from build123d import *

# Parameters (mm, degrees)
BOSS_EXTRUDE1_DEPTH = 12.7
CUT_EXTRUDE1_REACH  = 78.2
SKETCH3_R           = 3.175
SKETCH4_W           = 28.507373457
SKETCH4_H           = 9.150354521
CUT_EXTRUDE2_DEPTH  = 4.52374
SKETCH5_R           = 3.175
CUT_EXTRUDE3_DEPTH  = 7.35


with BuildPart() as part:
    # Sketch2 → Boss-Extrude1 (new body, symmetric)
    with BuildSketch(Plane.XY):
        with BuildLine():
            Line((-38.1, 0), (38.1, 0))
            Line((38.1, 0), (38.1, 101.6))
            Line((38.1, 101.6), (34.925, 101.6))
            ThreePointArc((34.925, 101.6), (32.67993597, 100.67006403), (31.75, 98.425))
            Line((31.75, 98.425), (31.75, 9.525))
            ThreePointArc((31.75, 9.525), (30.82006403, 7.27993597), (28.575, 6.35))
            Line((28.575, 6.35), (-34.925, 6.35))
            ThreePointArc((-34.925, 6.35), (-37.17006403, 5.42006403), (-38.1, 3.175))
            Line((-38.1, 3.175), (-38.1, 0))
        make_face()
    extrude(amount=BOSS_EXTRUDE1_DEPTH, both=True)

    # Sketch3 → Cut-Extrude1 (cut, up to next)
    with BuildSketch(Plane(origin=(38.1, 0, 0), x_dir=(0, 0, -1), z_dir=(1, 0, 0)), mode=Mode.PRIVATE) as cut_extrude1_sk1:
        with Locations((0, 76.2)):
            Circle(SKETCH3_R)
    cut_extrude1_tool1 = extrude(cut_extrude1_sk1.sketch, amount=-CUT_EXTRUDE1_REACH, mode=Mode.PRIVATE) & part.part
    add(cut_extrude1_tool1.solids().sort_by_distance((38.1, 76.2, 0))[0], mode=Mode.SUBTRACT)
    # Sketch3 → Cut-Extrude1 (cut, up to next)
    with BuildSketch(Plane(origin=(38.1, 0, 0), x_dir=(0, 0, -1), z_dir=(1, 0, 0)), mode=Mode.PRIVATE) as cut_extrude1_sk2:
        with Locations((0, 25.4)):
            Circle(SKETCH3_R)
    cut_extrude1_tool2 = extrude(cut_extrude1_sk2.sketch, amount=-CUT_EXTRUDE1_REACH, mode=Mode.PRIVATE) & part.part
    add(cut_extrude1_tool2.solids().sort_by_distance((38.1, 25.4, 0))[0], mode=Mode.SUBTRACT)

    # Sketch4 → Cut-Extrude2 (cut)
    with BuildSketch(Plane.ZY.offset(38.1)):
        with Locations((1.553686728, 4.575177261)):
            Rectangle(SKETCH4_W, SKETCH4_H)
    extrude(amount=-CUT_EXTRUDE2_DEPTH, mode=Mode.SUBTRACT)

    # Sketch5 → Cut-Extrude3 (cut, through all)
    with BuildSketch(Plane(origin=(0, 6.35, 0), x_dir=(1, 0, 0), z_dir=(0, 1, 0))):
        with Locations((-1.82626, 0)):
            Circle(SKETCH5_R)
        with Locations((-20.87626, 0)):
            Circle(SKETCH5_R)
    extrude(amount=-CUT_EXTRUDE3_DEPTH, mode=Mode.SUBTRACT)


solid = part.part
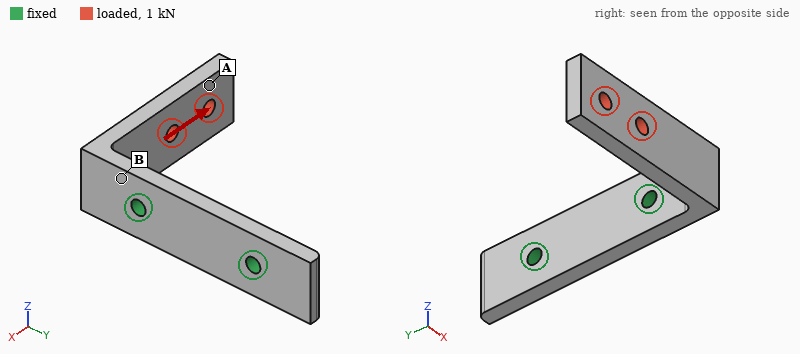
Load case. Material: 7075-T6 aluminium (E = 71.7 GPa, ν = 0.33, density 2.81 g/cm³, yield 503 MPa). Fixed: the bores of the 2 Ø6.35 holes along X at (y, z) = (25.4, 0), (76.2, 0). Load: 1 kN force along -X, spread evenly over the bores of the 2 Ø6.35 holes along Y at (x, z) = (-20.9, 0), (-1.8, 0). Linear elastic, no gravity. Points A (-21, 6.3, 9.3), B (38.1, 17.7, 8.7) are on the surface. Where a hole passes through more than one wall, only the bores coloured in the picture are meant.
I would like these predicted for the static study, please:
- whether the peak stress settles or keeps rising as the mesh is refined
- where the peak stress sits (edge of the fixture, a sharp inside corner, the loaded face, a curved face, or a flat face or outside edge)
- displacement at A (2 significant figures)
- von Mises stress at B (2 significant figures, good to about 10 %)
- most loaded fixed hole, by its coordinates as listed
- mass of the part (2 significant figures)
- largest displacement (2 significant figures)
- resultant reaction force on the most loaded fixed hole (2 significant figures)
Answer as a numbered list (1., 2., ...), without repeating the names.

1. keeps rising
2. edge of the fixture
3. 0.33 mm
4. 71 MPa
5. (25.4, 0)
6. 73 g
7. 0.42 mm
8. 1.0 kN
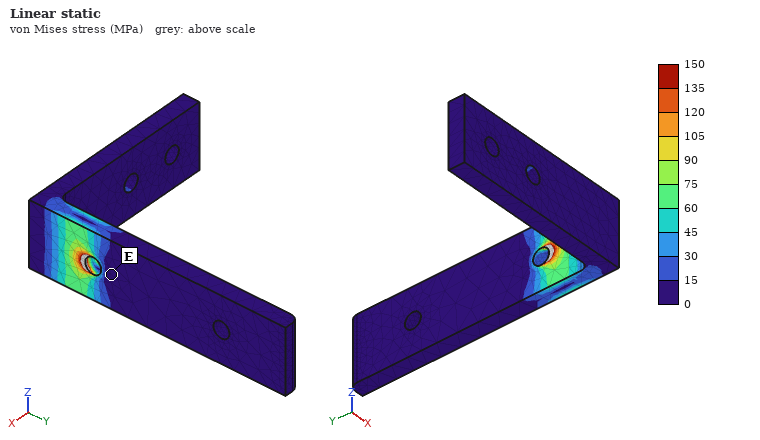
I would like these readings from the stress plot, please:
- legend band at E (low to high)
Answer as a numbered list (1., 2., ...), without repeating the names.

1. 0 to 15 MPa
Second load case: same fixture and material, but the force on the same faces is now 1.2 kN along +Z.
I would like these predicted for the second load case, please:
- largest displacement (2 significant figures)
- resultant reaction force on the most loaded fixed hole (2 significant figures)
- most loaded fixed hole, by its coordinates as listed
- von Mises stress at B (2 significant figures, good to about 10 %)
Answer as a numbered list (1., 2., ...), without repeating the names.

1. 1.4 mm
2. 1.5 kN
3. (25.4, 0)
4. 190 MPa
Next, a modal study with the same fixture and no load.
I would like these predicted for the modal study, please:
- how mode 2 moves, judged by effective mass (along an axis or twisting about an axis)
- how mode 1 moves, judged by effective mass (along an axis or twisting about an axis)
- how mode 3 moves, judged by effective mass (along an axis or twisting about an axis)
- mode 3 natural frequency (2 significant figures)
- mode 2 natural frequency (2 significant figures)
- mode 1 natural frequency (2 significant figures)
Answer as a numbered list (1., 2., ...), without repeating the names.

1. along Z
2. along Y
3. along X
4. 3600 Hz
5. 1200 Hz
6. 790 Hz
